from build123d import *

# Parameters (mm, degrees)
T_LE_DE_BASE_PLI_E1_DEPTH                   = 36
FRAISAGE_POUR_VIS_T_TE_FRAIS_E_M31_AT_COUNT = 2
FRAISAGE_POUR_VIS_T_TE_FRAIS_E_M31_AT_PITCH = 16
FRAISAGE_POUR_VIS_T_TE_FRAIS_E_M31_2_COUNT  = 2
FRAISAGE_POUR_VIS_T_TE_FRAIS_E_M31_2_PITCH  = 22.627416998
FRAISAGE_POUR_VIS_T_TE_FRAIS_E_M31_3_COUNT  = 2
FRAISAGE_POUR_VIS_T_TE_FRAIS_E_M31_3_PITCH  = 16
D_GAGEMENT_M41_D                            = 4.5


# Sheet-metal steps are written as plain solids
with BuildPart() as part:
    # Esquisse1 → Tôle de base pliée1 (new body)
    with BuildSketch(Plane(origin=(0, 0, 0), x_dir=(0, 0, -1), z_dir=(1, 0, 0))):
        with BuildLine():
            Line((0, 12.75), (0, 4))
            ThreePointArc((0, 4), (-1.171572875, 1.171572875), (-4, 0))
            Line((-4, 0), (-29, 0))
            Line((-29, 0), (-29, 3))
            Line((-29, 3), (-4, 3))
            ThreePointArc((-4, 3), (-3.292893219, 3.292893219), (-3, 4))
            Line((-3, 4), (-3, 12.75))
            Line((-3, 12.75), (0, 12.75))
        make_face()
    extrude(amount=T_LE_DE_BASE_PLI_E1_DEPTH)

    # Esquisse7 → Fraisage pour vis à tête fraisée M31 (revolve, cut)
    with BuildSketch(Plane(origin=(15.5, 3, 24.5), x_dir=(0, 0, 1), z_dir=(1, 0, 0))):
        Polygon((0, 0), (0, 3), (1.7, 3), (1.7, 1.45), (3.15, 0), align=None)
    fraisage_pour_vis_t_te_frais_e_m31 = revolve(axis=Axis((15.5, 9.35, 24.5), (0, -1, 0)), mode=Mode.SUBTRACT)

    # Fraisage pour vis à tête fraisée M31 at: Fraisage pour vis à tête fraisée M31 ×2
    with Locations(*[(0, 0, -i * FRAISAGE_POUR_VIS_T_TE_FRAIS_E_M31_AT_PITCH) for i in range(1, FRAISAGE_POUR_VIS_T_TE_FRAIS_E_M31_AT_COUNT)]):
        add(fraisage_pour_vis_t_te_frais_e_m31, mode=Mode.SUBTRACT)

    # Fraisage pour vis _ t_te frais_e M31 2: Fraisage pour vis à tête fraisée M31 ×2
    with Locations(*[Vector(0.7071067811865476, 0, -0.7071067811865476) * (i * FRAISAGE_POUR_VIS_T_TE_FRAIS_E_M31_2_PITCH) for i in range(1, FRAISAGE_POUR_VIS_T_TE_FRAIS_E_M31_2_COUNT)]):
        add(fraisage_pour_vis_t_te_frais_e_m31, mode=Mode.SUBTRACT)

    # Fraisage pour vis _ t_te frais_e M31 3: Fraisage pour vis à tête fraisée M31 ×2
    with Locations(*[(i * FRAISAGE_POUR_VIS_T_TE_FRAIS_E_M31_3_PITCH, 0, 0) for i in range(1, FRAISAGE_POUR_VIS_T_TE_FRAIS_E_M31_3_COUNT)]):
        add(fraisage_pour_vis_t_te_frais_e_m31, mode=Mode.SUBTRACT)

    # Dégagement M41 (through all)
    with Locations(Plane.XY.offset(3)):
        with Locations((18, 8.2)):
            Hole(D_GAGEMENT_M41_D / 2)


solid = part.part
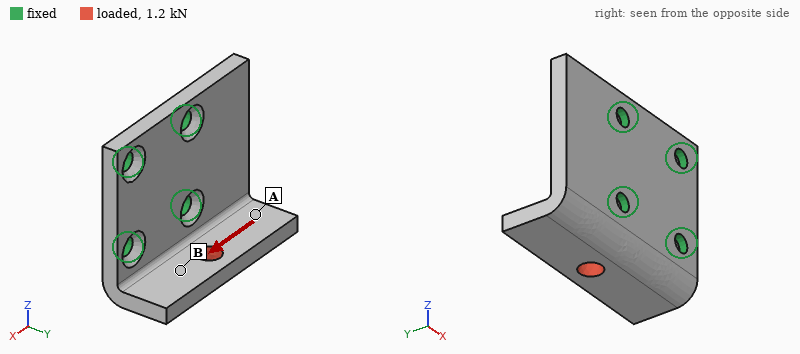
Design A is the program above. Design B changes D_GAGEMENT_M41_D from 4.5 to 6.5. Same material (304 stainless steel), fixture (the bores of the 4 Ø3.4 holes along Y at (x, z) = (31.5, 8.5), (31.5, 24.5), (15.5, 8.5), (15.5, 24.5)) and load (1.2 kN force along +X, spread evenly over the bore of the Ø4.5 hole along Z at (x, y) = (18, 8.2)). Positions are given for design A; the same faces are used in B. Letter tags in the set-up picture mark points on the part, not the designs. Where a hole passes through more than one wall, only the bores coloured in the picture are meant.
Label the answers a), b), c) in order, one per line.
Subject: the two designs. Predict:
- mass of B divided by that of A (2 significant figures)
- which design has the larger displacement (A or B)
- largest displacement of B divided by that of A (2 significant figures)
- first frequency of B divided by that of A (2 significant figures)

a) 0.99
b) B
c) 1.1
d) 1.0
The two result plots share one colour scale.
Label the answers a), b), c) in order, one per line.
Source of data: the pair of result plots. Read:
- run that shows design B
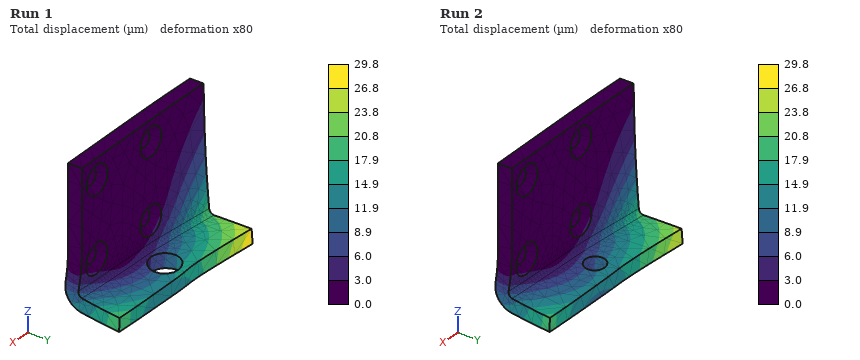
a) Run 1
